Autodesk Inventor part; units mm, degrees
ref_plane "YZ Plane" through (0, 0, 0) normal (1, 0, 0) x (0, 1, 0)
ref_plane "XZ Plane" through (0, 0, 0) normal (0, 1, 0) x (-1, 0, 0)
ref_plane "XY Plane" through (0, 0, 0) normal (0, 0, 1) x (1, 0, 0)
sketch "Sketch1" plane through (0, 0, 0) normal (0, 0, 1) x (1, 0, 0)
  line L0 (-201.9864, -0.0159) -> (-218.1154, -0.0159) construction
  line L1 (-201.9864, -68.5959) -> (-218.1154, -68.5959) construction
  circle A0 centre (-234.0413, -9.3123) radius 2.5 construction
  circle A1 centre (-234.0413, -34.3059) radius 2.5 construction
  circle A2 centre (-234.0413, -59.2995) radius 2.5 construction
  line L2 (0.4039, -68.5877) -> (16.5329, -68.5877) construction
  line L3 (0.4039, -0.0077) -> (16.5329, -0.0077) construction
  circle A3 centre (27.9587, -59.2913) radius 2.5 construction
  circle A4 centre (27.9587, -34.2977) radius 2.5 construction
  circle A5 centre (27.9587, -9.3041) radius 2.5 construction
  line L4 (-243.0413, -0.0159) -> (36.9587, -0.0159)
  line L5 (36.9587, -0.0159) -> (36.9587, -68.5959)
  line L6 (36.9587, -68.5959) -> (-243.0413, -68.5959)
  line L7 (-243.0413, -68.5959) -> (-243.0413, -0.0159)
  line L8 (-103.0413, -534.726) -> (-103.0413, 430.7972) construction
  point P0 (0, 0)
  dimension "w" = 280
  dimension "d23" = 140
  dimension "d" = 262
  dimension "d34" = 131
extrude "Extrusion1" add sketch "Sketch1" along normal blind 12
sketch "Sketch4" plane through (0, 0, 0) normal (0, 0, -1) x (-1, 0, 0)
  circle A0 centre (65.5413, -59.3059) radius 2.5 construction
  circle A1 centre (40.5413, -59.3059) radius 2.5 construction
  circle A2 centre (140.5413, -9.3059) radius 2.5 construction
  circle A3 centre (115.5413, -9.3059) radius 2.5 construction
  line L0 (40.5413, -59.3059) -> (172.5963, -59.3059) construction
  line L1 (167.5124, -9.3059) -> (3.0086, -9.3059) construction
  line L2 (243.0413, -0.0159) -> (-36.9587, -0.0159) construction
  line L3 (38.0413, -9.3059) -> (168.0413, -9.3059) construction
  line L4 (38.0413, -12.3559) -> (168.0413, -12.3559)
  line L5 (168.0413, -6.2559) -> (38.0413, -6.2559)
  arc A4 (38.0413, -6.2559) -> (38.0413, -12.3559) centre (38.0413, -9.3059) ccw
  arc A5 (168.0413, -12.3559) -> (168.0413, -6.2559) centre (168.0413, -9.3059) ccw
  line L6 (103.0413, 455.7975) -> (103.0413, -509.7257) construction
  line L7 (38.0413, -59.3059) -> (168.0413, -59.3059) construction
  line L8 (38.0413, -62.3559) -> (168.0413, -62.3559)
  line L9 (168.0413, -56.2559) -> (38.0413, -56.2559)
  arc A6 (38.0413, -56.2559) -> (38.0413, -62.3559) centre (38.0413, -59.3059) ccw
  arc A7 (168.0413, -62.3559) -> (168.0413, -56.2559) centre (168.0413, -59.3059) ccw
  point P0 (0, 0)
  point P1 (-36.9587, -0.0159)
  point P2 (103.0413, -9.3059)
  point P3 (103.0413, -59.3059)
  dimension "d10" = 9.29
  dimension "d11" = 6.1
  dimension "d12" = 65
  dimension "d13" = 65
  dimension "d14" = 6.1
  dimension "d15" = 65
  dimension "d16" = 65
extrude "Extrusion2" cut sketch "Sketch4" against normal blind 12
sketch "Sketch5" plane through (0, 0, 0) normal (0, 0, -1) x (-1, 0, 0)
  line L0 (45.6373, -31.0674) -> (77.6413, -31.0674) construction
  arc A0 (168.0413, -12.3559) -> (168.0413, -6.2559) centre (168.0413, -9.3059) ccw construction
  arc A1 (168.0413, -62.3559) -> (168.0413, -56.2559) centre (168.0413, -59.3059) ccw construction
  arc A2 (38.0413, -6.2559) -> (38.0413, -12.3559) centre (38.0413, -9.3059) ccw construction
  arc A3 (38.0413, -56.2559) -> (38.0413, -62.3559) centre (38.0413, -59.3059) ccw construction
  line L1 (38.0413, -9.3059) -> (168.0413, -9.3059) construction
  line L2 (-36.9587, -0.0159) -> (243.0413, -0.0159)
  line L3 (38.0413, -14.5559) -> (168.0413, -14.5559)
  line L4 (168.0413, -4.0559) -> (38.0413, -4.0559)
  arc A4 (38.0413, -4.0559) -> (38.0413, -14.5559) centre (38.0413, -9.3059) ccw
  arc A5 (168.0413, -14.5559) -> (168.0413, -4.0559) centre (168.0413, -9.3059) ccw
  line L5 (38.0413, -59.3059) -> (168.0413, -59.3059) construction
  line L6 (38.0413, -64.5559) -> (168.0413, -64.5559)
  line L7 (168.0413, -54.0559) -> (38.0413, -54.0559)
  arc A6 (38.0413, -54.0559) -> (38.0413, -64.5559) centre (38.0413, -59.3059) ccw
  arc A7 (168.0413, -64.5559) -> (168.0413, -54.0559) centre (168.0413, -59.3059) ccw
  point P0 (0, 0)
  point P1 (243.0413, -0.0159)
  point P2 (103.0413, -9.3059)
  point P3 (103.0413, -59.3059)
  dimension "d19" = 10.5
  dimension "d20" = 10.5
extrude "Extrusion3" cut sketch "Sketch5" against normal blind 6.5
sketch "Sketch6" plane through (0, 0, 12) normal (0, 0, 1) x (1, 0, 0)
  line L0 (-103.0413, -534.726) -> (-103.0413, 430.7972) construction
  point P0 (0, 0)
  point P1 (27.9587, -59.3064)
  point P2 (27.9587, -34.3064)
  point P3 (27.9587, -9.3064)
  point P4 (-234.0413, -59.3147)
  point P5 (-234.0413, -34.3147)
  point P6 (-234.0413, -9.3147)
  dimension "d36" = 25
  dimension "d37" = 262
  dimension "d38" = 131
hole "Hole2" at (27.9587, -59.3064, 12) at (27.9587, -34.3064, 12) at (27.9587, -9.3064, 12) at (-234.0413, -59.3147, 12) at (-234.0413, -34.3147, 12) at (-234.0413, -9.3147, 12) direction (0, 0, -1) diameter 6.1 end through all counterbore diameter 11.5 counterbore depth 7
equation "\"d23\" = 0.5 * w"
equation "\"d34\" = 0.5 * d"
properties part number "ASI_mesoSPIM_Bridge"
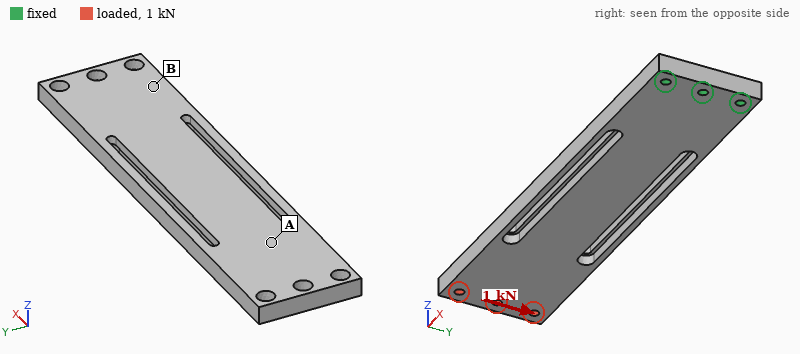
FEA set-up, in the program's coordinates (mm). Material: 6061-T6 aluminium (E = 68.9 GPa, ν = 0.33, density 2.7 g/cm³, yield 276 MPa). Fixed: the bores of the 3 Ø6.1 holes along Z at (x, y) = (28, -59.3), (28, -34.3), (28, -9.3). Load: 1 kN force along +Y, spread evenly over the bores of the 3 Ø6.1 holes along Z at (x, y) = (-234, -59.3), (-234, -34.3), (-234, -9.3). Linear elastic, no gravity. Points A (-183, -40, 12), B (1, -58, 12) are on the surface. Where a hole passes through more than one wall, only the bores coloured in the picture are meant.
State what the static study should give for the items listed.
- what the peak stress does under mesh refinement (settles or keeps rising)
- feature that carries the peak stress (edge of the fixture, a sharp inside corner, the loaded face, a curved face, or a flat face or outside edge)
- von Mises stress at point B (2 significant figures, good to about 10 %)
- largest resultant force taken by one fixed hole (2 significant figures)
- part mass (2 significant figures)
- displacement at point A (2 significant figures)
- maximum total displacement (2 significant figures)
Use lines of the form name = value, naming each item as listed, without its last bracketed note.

what the peak stress does under mesh refinement = keeps rising
feature that carries the peak stress = edge of the fixture
von Mises stress at point B = 13 MPa
largest resultant force taken by one fixed hole = 5.0 kN
part mass = 530 g
displacement at point A = 0.34 mm
maximum total displacement = 0.52 mm
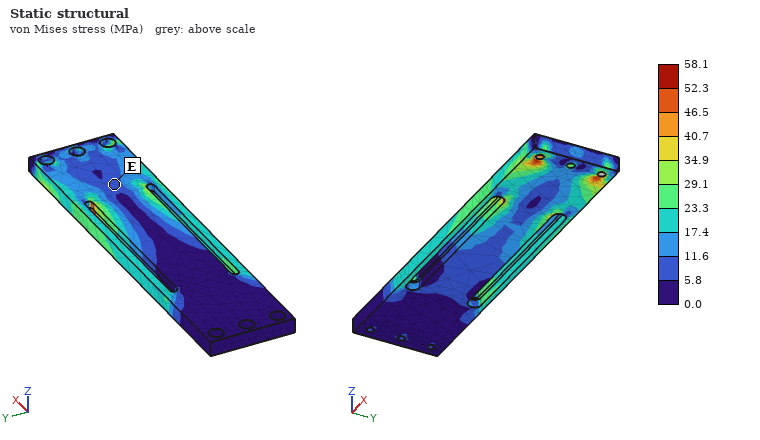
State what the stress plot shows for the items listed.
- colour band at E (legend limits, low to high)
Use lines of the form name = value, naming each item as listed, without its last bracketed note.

colour band at E = 5.8 to 11.6 MPa
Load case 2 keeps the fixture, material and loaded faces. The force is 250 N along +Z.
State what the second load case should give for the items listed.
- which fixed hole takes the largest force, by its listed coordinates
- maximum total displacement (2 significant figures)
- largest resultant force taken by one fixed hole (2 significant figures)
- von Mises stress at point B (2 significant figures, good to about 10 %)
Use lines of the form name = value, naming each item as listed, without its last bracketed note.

which fixed hole takes the largest force, by its listed coordinates = (28, -34.3)
maximum total displacement = 3.3 mm
largest resultant force taken by one fixed hole = 550 N
von Mises stress at point B = 35 MPa
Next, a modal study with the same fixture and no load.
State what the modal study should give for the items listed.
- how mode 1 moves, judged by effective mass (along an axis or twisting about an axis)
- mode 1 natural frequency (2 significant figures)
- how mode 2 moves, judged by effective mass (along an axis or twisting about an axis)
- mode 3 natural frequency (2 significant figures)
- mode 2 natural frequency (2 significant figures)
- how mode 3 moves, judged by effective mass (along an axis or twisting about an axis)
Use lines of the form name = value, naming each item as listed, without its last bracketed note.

how mode 1 moves, judged by effective mass = along Z
mode 1 natural frequency = 120 Hz
how mode 2 moves, judged by effective mass = along Y
mode 3 natural frequency = 750 Hz
mode 2 natural frequency = 590 Hz
how mode 3 moves, judged by effective mass = along Z
